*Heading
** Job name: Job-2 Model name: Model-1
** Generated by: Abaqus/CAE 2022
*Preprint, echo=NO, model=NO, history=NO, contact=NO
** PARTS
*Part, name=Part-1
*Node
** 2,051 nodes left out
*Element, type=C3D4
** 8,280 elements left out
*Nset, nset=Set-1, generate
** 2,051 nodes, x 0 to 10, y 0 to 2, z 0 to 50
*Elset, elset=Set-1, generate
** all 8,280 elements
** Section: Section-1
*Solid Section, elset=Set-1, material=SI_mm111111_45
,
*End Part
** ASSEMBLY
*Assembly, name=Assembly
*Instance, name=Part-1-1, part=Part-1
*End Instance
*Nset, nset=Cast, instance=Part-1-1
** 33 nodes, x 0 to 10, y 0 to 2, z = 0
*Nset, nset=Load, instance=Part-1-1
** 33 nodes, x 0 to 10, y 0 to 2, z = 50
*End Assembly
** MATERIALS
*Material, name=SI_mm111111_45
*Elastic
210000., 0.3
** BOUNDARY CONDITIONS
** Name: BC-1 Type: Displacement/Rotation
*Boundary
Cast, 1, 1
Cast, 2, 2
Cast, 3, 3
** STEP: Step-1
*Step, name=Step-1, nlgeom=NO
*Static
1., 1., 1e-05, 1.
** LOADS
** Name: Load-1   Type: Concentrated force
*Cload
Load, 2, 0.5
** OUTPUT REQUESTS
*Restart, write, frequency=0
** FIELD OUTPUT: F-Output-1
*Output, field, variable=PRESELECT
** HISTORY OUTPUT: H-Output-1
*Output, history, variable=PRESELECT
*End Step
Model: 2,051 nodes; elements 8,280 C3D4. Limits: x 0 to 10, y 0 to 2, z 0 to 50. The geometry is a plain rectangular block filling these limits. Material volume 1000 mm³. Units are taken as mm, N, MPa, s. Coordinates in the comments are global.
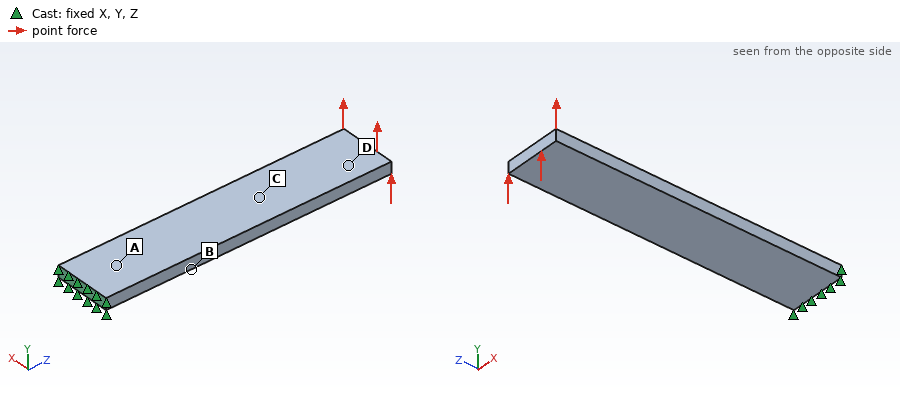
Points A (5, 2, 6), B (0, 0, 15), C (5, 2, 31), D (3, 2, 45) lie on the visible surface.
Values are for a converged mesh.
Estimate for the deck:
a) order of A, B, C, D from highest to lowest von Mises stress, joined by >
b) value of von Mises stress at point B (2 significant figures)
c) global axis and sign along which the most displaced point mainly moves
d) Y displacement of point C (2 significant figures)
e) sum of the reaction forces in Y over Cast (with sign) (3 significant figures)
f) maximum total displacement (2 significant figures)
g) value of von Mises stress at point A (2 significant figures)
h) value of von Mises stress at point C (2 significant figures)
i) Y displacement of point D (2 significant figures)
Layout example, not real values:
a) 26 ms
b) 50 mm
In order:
a) A > B > C > D
b) 87 MPa
c) +Y
d) 0.22 mm
e) -16.5 N
f) 0.48 mm
g) 100 MPa
h) 47 MPa
i) 0.41 mm
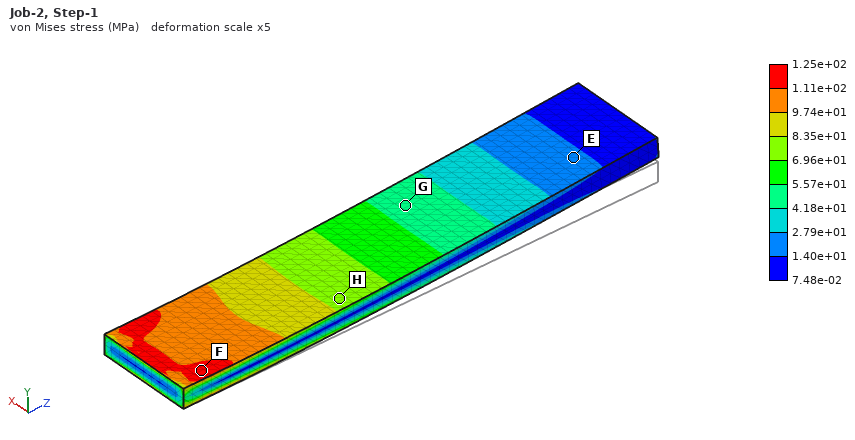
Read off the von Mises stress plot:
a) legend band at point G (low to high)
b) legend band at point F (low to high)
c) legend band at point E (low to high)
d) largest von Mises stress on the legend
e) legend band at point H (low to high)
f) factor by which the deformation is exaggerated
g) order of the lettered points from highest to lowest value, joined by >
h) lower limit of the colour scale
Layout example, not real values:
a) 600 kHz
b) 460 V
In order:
a) 4.18e+01 to 5.57e+01 MPa
b) 1.11e+02 to 1.25e+02 MPa
c) 1.40e+01 to 2.79e+01 MPa
d) 1.25e+02 MPa
e) 6.96e+01 to 8.35e+01 MPa
f) 5
g) F > H > G > E
h) 7.48e-02 MPa
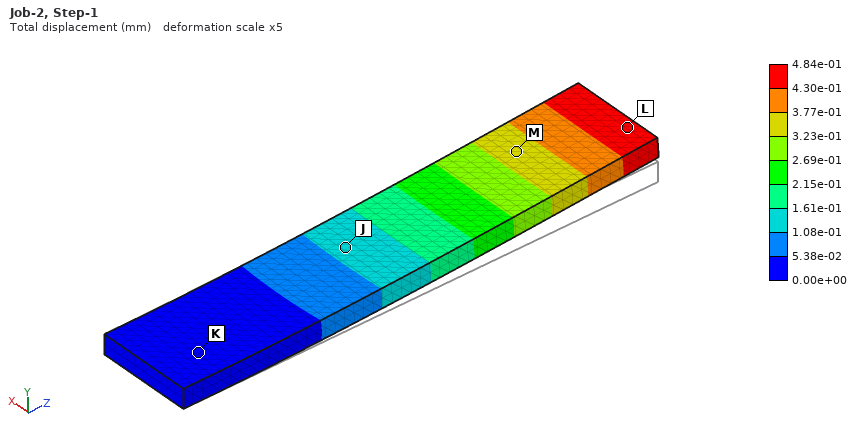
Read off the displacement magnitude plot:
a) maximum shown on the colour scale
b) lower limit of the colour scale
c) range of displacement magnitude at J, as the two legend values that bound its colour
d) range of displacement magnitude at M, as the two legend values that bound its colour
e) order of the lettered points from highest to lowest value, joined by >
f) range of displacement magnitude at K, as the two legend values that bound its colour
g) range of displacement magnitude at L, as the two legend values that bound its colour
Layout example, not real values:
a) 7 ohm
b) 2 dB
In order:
a) 4.84e-01 mm
b) 0.00e+00 mm
c) 1.08e-01 to 1.61e-01 mm
d) 3.23e-01 to 3.77e-01 mm
e) L > M > J > K
f) 0.00e+00 to 5.38e-02 mm
g) 4.30e-01 to 4.84e-01 mm
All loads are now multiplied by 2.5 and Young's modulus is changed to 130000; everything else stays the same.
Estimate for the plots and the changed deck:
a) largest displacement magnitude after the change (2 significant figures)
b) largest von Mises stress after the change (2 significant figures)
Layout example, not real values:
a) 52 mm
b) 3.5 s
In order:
a) 2.0 mm
b) 310 MPa
